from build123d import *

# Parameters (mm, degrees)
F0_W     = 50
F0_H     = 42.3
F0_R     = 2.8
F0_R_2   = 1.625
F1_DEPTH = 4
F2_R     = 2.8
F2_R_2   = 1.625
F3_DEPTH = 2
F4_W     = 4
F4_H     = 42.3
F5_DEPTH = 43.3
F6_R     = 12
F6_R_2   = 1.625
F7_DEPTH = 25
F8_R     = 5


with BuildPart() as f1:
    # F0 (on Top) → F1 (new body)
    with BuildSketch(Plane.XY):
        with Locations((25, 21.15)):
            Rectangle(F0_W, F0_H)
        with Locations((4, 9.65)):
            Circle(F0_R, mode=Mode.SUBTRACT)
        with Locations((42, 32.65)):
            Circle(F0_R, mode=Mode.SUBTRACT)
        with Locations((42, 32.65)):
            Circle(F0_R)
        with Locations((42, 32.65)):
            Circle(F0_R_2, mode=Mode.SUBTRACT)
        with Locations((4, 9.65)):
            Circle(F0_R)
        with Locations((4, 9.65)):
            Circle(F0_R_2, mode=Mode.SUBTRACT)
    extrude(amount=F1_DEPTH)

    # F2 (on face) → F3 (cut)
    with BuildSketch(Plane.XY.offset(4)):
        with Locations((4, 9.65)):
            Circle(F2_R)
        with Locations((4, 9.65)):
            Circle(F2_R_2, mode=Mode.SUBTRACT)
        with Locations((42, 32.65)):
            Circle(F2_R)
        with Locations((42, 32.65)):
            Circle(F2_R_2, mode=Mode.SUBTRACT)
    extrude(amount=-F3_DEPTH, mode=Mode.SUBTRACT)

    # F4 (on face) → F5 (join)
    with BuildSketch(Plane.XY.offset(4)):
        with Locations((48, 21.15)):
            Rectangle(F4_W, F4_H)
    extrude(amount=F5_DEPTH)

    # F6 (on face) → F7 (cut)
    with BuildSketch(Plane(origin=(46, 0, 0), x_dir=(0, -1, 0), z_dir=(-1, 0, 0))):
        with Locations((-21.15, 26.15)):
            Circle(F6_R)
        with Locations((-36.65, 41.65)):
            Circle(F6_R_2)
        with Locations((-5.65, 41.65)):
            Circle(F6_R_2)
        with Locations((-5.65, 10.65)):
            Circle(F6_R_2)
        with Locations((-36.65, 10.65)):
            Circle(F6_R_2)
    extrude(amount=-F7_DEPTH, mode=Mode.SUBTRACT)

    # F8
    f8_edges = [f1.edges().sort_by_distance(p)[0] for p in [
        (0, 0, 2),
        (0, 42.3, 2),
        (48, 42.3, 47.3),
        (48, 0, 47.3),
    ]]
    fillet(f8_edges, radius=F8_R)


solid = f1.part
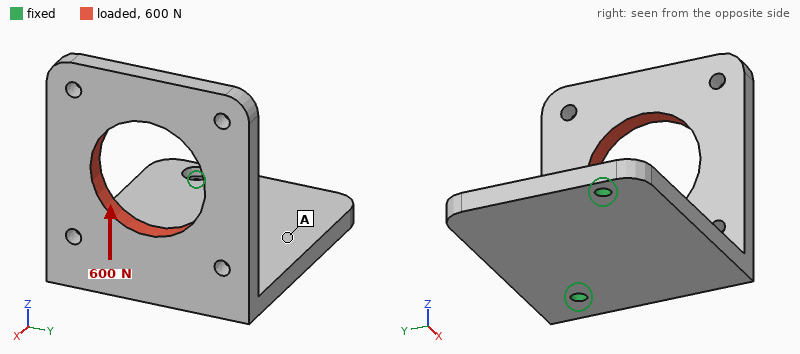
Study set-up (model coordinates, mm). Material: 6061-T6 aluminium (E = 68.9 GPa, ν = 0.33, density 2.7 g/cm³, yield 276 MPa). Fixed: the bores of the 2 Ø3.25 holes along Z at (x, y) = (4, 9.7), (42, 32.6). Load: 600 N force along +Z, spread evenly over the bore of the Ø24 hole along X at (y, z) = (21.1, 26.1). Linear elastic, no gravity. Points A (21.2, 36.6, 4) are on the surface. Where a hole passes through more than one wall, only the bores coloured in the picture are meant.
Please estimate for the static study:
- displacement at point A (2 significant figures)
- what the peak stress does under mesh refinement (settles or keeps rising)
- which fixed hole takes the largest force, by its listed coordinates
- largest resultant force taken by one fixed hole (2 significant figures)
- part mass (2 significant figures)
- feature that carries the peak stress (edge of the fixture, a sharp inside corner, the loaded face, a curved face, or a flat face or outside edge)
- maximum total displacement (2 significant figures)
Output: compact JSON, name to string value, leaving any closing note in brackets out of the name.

{"displacement at point A": "0.069 mm", "what the peak stress does under mesh refinement": "keeps rising", "which fixed hole takes the largest force, by its listed coordinates": "(42, 32.6)", "largest resultant force taken by one fixed hole": "580 N", "part mass": "37 g", "feature that carries the peak stress": "edge of the fixture", "maximum total displacement": "0.45 mm"}
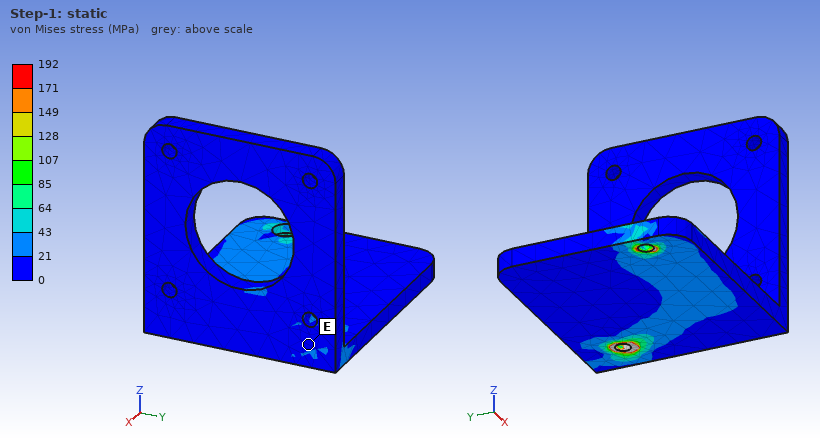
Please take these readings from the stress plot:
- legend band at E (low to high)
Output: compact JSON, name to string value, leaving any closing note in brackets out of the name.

{"legend band at E": "0 to 21 MPa"}
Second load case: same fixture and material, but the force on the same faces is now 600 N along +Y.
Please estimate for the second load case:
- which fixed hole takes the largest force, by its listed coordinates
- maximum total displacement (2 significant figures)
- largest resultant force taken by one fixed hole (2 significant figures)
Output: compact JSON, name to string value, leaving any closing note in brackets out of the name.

{"which fixed hole takes the largest force, by its listed coordinates": "(42, 32.6)", "maximum total displacement": "0.80 mm", "largest resultant force taken by one fixed hole": "620 N"}
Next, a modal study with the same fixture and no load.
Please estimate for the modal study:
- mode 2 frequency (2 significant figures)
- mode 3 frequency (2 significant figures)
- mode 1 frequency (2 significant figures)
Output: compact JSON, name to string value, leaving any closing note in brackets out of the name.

{"mode 2 frequency": "1400 Hz", "mode 3 frequency": "3100 Hz", "mode 1 frequency": "1000 Hz"}
